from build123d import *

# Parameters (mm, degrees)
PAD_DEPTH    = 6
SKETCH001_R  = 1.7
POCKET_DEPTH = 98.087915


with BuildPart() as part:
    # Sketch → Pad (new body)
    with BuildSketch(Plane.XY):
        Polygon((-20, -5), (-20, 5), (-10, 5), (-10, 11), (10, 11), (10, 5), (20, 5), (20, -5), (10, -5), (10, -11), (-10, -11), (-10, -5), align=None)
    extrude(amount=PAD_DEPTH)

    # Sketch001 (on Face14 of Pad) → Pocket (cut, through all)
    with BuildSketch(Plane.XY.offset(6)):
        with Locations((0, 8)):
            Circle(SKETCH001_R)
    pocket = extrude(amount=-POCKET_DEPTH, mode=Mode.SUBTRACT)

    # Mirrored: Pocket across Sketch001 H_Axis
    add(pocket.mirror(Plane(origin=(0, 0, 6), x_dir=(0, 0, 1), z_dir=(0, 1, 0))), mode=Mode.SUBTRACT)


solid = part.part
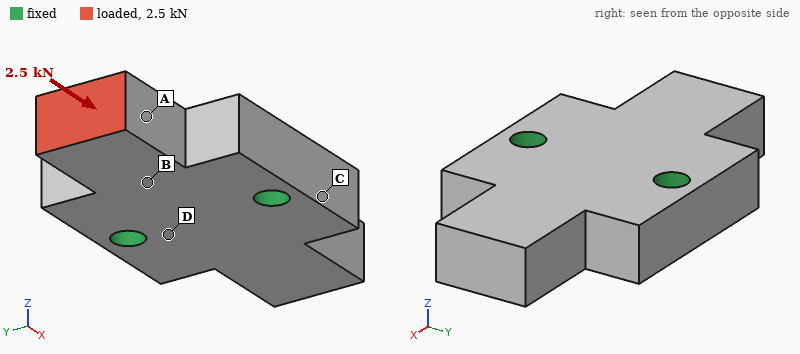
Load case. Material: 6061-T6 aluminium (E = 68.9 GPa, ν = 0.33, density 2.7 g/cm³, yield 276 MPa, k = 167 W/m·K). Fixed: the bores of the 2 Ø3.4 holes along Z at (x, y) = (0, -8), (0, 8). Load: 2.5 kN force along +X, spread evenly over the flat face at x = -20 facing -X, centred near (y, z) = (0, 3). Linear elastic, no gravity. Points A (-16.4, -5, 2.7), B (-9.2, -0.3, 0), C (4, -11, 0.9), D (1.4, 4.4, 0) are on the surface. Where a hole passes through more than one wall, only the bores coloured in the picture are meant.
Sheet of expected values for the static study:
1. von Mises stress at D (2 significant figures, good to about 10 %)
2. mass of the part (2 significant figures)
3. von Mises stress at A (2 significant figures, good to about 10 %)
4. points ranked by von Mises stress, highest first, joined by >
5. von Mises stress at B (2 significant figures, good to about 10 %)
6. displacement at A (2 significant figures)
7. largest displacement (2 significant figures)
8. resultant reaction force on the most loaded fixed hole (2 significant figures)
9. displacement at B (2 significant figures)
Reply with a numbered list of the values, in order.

1. 15 MPa
2. 10 g
3. 41 MPa
4. A > B > D > C
5. 28 MPa
6. 8.9 µm
7. 11 µm
8. 1.3 kN
9. 5.0 µm
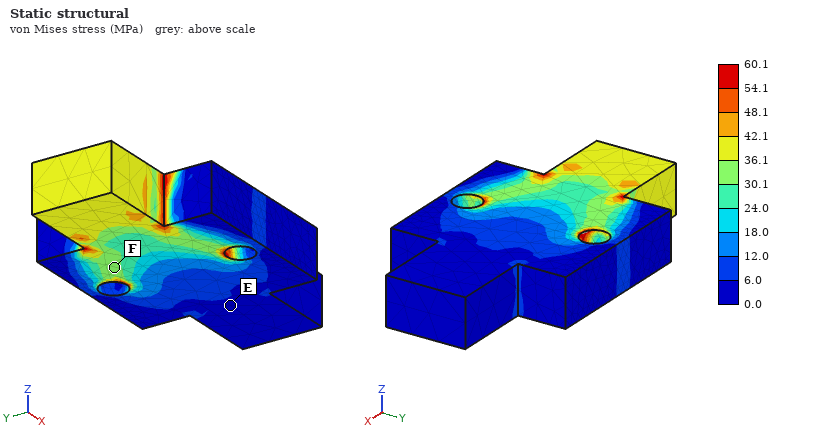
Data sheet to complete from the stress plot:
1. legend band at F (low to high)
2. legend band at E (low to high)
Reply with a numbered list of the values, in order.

1. 30.1 to 36.1 MPa
2. 0.0 to 6.0 MPa
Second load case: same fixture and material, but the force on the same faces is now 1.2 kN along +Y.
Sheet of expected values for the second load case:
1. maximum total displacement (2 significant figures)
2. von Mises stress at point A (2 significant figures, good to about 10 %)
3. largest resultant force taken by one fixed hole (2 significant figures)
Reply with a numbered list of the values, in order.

1. 44 µm
2. 46 MPa
3. 1.5 kN
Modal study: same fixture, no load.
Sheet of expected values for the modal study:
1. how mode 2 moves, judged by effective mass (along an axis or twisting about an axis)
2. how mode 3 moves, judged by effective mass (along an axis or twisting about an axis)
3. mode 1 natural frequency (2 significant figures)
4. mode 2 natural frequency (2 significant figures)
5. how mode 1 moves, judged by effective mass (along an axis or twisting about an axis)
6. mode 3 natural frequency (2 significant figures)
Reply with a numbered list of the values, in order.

1. along Z
2. twisting about Z
3. 13 kHz
4. 15 kHz
5. twisting about Y
6. 32 kHz
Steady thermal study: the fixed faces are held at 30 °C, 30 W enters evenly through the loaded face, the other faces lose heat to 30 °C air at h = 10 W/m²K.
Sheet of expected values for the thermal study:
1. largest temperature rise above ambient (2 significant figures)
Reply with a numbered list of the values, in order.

1. 48 K
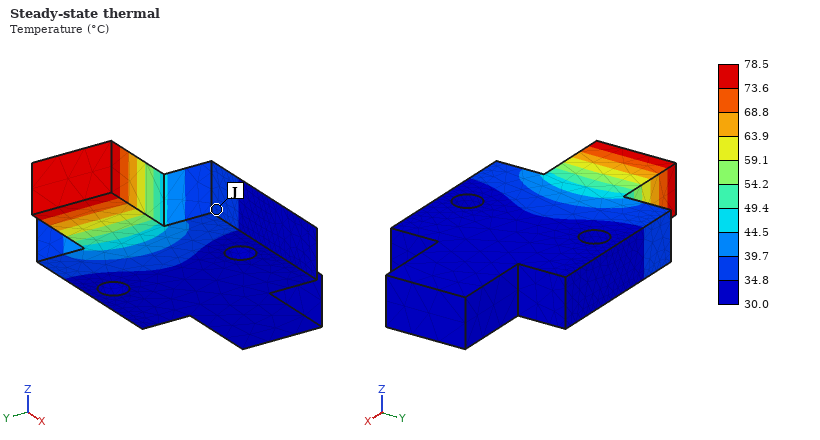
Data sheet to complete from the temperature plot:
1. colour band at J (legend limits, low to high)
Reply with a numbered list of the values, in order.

1. 34.8 to 39.7 °C
